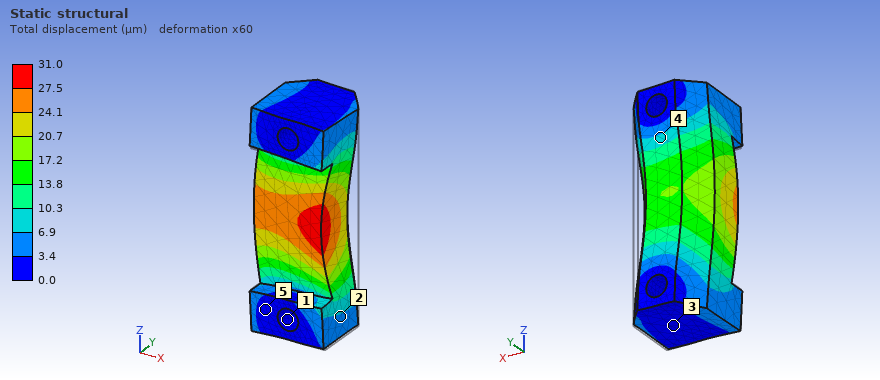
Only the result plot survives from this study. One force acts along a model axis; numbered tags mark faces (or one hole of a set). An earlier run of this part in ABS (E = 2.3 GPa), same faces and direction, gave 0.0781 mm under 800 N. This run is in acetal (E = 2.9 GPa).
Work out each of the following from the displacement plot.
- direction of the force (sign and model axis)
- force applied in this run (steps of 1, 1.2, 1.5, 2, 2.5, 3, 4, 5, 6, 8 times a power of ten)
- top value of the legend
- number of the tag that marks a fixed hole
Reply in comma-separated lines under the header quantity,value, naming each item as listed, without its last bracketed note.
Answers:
quantity,value
direction of the force,-X
force applied in this run,400 N
top value of the legend,31.0 µm
number of the tag that marks a fixed hole,1
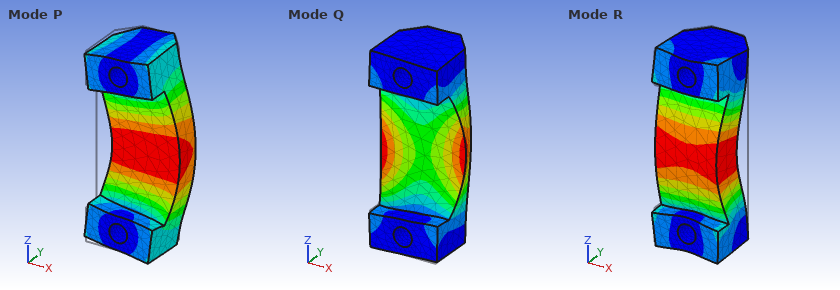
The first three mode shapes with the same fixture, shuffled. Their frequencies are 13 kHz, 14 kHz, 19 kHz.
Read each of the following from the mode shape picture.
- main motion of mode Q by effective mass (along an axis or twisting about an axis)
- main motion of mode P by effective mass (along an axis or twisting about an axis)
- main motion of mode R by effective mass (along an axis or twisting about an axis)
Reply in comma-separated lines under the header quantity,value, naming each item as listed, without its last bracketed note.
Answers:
quantity,value
main motion of mode Q by effective mass,twisting about Z
main motion of mode P by effective mass,along X
main motion of mode R by effective mass,along Y
